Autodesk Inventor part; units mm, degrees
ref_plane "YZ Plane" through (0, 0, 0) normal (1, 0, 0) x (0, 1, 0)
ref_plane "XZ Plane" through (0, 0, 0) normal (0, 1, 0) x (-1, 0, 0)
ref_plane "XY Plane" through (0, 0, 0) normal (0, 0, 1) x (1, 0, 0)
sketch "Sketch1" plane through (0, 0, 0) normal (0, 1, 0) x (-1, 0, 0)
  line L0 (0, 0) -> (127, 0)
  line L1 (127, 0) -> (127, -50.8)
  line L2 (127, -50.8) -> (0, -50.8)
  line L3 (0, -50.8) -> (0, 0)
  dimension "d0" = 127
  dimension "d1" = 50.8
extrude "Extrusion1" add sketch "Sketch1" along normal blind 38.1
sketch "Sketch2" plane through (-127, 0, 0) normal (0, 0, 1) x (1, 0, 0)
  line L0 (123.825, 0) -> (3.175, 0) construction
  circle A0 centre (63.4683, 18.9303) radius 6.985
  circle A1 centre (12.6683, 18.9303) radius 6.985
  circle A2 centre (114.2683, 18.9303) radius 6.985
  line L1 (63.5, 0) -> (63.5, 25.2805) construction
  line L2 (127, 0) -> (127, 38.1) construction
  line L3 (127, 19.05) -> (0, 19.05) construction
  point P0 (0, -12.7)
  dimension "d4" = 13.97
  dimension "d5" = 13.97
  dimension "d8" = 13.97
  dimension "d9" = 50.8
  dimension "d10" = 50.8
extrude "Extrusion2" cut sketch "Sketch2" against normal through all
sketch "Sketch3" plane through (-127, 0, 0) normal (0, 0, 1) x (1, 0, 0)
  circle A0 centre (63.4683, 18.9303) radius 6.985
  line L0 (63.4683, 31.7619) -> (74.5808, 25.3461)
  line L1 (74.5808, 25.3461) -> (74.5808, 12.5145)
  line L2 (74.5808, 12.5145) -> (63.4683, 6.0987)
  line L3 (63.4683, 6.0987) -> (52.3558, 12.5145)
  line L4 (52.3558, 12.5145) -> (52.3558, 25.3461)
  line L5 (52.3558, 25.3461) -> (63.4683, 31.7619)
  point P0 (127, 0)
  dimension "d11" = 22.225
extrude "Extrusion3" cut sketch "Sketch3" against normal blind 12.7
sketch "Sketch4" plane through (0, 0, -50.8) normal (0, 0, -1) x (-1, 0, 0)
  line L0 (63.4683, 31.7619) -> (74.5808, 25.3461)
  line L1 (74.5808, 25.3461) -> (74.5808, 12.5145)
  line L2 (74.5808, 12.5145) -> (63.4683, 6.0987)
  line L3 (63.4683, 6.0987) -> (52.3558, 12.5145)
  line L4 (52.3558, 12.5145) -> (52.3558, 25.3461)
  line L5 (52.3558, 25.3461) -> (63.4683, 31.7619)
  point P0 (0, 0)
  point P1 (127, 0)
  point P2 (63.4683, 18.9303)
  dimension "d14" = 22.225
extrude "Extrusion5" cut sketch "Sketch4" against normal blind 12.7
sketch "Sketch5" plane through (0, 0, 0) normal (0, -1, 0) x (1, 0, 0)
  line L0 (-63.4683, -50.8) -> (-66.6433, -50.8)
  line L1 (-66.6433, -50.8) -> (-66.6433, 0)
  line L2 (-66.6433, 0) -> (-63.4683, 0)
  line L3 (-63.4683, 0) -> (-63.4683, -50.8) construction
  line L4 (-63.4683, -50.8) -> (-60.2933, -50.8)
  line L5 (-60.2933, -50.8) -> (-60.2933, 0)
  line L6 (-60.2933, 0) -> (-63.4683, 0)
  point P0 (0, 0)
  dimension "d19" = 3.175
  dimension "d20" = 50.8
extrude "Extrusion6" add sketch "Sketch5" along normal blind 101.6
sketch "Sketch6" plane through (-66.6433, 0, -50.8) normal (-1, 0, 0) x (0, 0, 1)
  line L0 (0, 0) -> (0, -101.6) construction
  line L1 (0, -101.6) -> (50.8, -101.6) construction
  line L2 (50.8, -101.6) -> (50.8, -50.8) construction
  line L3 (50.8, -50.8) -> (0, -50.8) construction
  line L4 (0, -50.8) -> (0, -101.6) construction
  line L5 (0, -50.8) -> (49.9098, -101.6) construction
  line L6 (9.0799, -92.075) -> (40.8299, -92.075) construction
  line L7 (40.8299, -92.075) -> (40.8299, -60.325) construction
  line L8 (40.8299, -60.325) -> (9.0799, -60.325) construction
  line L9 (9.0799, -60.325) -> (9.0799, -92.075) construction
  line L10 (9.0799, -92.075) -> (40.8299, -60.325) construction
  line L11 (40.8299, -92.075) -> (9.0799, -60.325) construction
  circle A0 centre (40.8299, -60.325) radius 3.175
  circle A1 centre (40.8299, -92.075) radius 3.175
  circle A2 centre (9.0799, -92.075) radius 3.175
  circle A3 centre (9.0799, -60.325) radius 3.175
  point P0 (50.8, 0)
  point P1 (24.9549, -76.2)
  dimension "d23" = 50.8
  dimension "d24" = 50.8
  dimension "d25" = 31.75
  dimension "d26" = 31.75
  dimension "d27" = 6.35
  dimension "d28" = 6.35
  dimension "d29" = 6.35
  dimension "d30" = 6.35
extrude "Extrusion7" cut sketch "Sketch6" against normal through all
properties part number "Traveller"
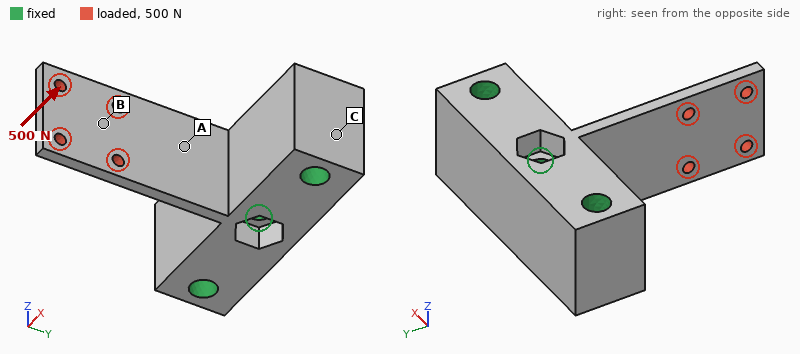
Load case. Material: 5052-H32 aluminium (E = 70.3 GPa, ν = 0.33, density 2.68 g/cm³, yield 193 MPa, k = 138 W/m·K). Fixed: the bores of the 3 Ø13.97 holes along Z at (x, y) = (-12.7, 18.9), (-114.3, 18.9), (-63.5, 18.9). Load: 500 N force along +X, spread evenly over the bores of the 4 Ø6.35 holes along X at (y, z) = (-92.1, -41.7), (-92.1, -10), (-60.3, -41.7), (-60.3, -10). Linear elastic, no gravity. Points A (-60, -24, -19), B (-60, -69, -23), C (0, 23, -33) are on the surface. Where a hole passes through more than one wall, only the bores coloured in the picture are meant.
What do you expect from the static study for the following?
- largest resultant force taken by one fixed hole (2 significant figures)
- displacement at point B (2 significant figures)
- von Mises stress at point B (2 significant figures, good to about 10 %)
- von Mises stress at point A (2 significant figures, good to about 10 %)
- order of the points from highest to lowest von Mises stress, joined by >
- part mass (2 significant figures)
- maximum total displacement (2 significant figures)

610 N
0.86 mm
20 MPa
70 MPa
A > B > C
660 g
1.5 mm
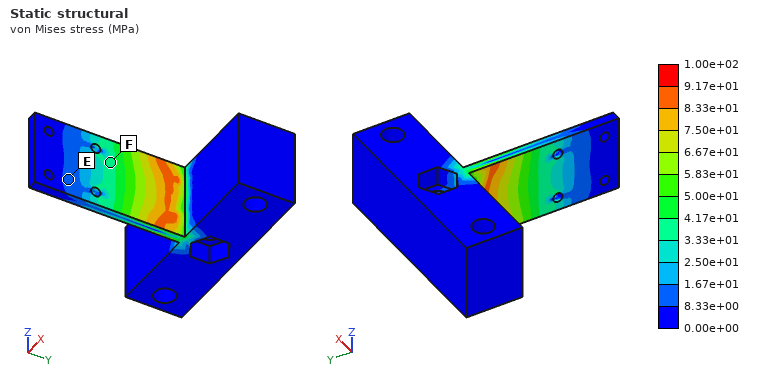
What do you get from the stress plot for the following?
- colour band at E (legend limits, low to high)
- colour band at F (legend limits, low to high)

8.33e+00 to 1.67e+01 MPa
3.33e+01 to 4.17e+01 MPa
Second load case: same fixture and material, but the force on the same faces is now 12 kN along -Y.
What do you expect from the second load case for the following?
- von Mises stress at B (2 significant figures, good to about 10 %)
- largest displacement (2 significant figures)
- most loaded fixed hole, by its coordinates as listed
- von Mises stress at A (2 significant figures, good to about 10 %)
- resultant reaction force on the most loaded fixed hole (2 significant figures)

26 MPa
55 µm
(-63.5, 18.9)
39 MPa
10 kN
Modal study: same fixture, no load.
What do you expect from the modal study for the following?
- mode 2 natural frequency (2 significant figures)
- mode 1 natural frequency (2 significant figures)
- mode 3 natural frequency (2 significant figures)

2100 Hz
510 Hz
2700 Hz
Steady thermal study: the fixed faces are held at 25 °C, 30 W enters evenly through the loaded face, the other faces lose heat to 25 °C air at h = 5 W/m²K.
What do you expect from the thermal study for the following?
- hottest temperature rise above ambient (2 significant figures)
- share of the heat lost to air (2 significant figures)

56 K
6.8 %
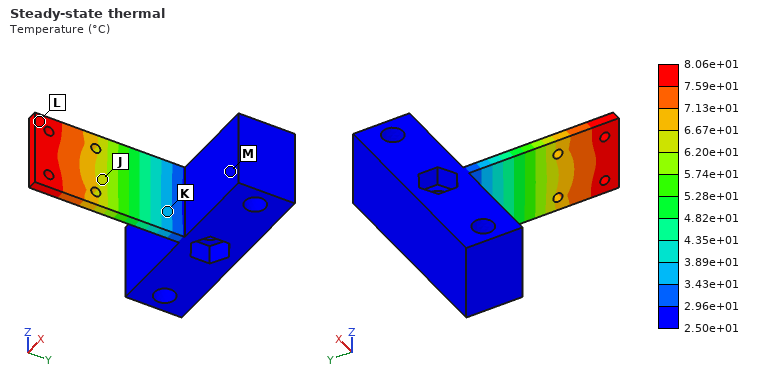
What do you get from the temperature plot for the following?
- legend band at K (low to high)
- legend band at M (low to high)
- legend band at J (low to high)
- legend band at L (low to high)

3.43e+01 to 3.89e+01 °C
2.50e+01 to 2.96e+01 °C
6.20e+01 to 6.67e+01 °C
7.59e+01 to 8.06e+01 °C
